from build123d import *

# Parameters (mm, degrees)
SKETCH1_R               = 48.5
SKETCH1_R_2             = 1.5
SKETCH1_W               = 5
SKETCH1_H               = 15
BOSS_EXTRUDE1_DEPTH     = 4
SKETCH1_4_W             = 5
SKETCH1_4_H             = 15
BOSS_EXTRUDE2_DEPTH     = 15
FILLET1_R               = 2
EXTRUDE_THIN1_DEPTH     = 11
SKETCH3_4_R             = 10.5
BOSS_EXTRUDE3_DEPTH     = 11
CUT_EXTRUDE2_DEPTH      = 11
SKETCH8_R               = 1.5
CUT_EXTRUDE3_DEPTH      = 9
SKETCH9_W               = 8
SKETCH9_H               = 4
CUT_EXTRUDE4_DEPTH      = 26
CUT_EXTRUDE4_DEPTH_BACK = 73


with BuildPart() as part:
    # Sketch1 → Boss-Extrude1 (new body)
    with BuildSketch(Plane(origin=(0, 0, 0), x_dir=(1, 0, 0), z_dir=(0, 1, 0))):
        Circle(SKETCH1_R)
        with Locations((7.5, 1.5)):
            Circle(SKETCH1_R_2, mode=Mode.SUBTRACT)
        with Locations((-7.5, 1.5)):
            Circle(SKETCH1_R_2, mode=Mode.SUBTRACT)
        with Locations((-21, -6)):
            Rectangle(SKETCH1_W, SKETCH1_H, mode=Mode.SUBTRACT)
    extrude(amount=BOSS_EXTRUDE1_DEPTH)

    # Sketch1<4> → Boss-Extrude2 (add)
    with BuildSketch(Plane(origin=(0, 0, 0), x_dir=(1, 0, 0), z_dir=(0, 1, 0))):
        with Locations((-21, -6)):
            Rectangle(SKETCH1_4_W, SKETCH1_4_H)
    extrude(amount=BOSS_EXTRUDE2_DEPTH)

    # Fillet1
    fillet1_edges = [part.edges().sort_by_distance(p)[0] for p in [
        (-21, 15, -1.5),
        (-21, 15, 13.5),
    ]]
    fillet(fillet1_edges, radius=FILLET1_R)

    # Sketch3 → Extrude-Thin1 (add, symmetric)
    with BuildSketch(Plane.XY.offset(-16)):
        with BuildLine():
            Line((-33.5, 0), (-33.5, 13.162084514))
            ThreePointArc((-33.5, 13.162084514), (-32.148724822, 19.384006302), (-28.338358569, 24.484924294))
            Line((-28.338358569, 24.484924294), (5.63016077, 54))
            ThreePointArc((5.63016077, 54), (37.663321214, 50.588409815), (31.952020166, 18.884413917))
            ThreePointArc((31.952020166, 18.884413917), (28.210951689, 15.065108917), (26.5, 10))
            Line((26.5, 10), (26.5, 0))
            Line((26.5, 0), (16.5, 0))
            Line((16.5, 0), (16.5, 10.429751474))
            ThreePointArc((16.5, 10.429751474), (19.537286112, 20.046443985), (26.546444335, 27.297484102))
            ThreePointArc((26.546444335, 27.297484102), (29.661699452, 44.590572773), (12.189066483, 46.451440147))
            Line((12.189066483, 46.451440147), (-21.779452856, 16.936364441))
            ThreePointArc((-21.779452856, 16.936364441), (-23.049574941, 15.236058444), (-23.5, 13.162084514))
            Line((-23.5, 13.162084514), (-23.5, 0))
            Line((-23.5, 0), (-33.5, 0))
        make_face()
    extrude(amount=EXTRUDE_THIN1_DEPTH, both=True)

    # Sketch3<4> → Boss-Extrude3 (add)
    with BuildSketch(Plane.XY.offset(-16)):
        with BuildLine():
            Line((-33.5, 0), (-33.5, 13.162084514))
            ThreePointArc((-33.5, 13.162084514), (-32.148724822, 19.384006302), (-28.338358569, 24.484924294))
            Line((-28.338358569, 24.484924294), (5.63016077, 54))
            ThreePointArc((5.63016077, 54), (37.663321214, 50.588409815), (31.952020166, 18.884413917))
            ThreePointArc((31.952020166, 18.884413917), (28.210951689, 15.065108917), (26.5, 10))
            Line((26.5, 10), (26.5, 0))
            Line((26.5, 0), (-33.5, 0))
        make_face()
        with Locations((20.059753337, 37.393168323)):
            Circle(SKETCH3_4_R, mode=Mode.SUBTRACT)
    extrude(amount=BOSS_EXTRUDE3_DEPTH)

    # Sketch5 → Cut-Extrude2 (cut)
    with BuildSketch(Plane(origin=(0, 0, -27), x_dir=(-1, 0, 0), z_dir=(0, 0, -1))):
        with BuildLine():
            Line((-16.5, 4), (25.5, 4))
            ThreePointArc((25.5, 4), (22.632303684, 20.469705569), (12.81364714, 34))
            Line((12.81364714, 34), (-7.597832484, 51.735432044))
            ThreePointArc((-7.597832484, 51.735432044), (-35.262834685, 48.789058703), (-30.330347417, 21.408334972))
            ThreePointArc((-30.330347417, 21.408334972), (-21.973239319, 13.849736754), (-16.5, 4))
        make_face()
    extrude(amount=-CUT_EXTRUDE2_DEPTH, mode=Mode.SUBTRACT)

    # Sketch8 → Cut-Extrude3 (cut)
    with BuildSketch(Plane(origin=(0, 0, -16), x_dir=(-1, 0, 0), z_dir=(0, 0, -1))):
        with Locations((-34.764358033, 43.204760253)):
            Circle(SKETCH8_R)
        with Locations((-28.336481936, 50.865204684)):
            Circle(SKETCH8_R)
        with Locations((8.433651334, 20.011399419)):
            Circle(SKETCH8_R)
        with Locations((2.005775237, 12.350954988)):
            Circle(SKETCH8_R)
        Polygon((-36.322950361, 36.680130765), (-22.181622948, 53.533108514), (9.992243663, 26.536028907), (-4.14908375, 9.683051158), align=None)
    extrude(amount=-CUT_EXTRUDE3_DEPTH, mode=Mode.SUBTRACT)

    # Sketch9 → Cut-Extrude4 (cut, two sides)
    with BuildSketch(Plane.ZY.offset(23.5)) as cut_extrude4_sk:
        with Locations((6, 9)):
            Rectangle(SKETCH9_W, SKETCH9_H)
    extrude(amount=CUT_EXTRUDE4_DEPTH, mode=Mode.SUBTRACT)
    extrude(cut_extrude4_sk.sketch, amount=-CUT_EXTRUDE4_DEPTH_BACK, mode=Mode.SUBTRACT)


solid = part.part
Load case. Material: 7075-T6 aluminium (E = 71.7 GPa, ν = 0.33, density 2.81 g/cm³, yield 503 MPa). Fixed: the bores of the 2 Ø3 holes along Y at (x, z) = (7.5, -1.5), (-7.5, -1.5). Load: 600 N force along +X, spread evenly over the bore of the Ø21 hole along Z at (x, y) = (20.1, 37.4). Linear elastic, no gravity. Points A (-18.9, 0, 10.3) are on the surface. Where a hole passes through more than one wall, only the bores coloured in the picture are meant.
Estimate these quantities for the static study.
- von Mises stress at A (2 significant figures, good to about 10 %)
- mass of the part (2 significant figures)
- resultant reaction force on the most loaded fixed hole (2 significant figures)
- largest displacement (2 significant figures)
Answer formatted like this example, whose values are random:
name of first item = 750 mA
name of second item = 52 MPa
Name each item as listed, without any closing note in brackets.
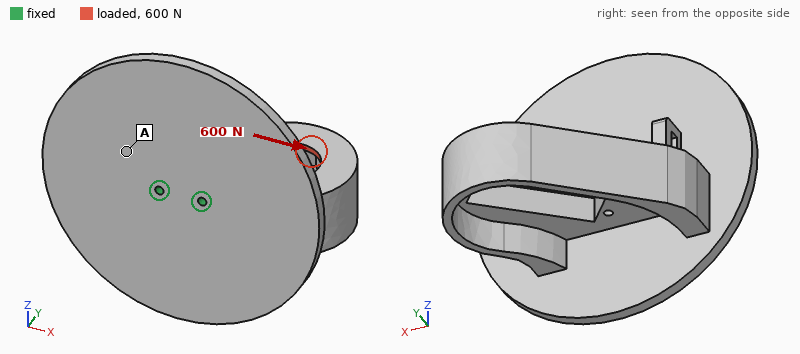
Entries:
von Mises stress at A = 7.6 MPa
mass of the part = 170 g
resultant reaction force on the most loaded fixed hole = 1.2 kN
largest displacement = 85 µm
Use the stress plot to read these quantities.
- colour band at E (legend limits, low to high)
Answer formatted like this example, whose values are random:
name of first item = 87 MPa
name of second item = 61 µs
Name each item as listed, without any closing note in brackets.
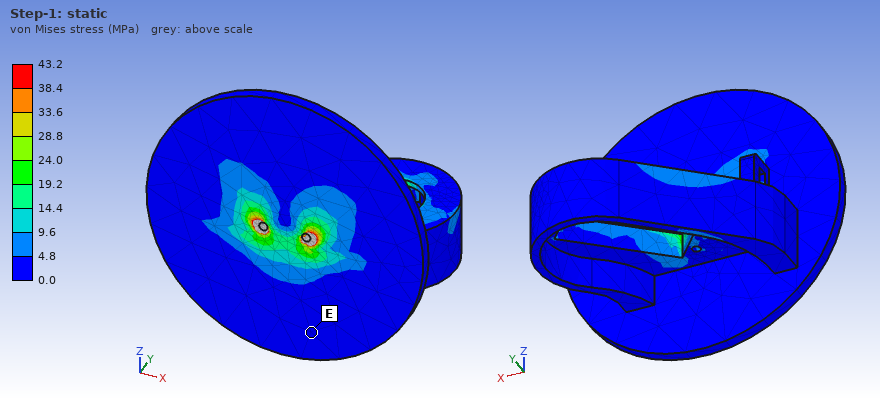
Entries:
colour band at E = 0.0 to 4.8 MPa
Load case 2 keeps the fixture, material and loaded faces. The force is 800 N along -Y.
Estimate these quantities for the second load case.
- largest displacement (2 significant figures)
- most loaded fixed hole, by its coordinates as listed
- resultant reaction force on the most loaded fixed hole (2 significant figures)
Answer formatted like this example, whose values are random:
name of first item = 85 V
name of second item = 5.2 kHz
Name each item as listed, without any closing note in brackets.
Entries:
largest displacement = 80 µm
most loaded fixed hole, by its coordinates as listed = (7.5, -1.5)
resultant reaction force on the most loaded fixed hole = 1.2 kN
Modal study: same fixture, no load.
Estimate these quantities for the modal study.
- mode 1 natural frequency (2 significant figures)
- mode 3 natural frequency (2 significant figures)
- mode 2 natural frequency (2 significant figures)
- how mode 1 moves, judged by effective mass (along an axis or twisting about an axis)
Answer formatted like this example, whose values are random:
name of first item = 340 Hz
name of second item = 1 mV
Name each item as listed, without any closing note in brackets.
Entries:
mode 1 natural frequency = 770 Hz
mode 3 natural frequency = 1700 Hz
mode 2 natural frequency = 1600 Hz
how mode 1 moves, judged by effective mass = along Z
